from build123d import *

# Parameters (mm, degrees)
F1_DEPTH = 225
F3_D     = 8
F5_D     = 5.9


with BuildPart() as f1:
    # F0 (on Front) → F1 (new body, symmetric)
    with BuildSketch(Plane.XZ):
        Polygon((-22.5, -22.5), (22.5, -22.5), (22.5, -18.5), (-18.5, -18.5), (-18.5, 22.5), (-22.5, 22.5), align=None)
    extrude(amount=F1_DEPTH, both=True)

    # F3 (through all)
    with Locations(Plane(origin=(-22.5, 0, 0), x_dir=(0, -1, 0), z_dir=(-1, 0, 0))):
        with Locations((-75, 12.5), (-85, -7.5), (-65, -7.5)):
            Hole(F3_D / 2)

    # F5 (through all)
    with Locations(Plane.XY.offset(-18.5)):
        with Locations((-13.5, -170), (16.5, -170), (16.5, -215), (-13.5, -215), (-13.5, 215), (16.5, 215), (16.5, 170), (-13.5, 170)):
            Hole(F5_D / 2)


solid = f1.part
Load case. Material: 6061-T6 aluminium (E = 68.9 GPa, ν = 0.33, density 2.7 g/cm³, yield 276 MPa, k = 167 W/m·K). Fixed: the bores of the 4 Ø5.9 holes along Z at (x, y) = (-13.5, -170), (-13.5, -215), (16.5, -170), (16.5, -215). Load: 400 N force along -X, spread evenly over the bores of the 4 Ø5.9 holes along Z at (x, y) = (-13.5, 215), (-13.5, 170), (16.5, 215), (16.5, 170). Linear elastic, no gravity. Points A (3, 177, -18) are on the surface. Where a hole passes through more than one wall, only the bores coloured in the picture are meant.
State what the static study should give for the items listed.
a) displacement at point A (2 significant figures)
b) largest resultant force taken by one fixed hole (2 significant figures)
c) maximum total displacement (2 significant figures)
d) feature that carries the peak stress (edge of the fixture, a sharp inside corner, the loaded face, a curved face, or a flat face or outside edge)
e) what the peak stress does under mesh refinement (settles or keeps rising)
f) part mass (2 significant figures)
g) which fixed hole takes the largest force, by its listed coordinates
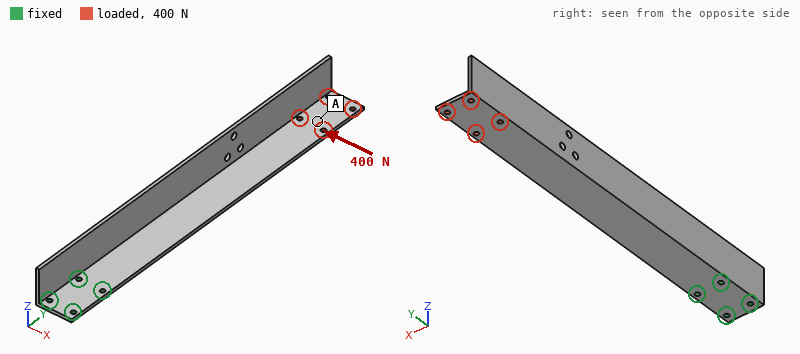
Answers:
2.4 mm
4.1 kN
2.9 mm
edge of the fixture
keeps rising
410 g
(16.5, -170)
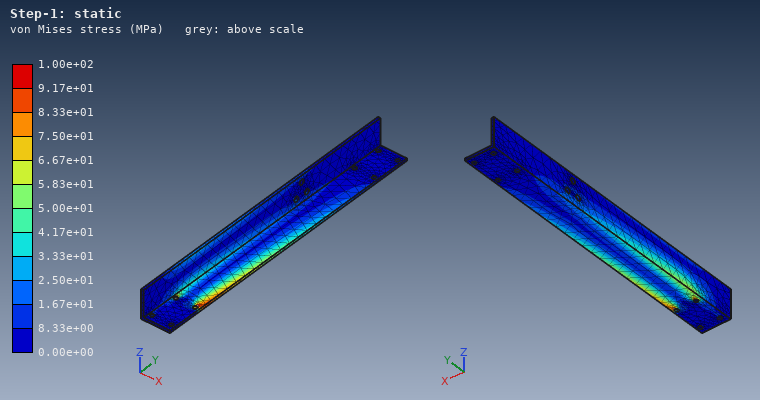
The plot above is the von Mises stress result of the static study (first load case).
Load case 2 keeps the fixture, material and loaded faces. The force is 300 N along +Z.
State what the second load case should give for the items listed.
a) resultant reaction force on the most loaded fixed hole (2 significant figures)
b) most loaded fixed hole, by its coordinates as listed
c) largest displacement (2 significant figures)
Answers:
3.0 kN
(-13.5, -170)
4.8 mm
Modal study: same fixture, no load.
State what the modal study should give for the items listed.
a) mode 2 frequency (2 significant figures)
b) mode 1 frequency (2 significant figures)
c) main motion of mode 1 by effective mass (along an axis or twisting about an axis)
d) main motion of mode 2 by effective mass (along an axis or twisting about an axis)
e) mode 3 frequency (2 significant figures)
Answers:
170 Hz
140 Hz
along Z
along X
340 Hz
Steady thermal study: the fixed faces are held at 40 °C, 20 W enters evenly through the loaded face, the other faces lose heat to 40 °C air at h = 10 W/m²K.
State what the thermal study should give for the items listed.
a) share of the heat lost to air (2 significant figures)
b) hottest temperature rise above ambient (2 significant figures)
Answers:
79 %
58 K
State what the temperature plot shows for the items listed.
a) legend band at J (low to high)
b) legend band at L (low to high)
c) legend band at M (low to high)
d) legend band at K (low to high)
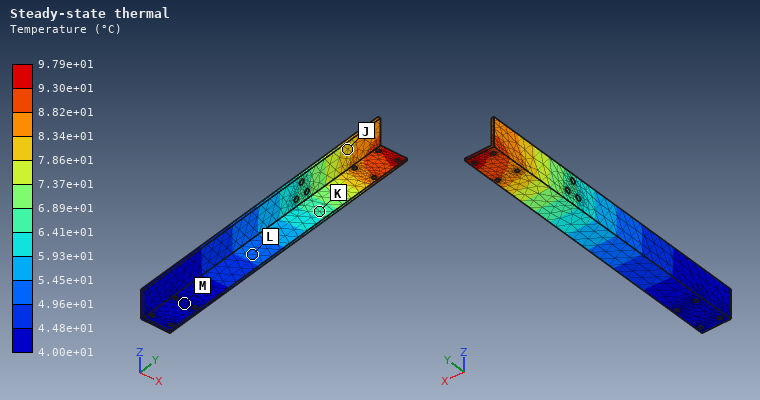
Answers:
7.86e+01 to 8.34e+01 °C
4.96e+01 to 5.45e+01 °C
4.00e+01 to 4.48e+01 °C
6.41e+01 to 6.89e+01 °C
